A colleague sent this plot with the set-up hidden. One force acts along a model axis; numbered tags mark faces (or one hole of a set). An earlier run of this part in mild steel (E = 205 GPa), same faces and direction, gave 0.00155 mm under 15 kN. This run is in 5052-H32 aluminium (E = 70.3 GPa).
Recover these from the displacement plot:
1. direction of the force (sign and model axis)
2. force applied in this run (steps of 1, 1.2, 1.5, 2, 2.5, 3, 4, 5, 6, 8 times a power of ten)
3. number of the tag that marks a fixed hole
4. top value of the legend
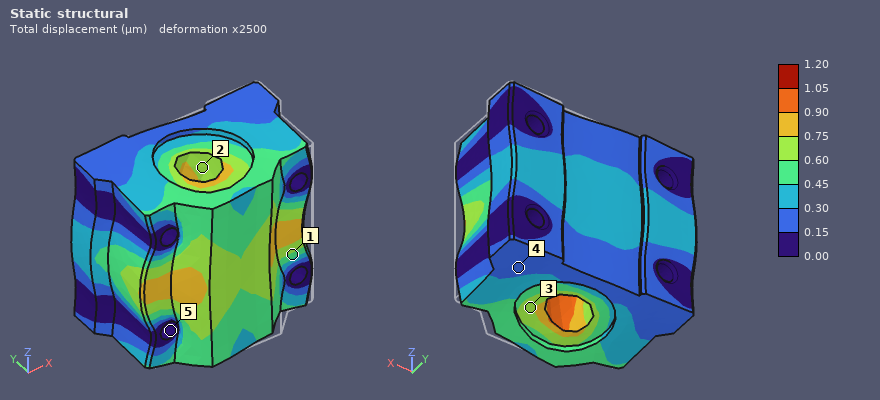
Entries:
-X
4 kN
5
1.20 µm
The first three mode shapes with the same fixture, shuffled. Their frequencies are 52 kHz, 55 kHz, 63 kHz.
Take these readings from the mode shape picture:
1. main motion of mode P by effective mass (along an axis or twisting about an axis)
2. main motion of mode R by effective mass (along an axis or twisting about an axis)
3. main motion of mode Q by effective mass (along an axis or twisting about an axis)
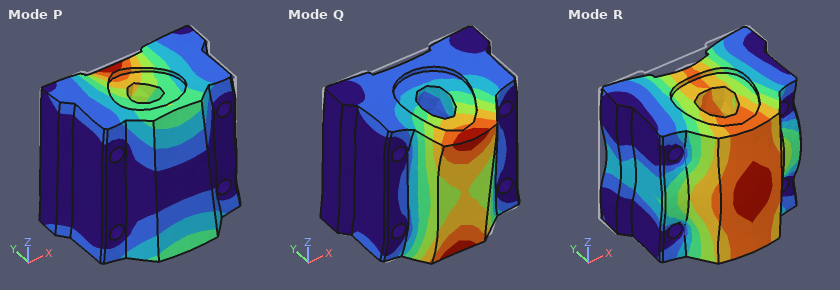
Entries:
along Z
along Y
along Z
